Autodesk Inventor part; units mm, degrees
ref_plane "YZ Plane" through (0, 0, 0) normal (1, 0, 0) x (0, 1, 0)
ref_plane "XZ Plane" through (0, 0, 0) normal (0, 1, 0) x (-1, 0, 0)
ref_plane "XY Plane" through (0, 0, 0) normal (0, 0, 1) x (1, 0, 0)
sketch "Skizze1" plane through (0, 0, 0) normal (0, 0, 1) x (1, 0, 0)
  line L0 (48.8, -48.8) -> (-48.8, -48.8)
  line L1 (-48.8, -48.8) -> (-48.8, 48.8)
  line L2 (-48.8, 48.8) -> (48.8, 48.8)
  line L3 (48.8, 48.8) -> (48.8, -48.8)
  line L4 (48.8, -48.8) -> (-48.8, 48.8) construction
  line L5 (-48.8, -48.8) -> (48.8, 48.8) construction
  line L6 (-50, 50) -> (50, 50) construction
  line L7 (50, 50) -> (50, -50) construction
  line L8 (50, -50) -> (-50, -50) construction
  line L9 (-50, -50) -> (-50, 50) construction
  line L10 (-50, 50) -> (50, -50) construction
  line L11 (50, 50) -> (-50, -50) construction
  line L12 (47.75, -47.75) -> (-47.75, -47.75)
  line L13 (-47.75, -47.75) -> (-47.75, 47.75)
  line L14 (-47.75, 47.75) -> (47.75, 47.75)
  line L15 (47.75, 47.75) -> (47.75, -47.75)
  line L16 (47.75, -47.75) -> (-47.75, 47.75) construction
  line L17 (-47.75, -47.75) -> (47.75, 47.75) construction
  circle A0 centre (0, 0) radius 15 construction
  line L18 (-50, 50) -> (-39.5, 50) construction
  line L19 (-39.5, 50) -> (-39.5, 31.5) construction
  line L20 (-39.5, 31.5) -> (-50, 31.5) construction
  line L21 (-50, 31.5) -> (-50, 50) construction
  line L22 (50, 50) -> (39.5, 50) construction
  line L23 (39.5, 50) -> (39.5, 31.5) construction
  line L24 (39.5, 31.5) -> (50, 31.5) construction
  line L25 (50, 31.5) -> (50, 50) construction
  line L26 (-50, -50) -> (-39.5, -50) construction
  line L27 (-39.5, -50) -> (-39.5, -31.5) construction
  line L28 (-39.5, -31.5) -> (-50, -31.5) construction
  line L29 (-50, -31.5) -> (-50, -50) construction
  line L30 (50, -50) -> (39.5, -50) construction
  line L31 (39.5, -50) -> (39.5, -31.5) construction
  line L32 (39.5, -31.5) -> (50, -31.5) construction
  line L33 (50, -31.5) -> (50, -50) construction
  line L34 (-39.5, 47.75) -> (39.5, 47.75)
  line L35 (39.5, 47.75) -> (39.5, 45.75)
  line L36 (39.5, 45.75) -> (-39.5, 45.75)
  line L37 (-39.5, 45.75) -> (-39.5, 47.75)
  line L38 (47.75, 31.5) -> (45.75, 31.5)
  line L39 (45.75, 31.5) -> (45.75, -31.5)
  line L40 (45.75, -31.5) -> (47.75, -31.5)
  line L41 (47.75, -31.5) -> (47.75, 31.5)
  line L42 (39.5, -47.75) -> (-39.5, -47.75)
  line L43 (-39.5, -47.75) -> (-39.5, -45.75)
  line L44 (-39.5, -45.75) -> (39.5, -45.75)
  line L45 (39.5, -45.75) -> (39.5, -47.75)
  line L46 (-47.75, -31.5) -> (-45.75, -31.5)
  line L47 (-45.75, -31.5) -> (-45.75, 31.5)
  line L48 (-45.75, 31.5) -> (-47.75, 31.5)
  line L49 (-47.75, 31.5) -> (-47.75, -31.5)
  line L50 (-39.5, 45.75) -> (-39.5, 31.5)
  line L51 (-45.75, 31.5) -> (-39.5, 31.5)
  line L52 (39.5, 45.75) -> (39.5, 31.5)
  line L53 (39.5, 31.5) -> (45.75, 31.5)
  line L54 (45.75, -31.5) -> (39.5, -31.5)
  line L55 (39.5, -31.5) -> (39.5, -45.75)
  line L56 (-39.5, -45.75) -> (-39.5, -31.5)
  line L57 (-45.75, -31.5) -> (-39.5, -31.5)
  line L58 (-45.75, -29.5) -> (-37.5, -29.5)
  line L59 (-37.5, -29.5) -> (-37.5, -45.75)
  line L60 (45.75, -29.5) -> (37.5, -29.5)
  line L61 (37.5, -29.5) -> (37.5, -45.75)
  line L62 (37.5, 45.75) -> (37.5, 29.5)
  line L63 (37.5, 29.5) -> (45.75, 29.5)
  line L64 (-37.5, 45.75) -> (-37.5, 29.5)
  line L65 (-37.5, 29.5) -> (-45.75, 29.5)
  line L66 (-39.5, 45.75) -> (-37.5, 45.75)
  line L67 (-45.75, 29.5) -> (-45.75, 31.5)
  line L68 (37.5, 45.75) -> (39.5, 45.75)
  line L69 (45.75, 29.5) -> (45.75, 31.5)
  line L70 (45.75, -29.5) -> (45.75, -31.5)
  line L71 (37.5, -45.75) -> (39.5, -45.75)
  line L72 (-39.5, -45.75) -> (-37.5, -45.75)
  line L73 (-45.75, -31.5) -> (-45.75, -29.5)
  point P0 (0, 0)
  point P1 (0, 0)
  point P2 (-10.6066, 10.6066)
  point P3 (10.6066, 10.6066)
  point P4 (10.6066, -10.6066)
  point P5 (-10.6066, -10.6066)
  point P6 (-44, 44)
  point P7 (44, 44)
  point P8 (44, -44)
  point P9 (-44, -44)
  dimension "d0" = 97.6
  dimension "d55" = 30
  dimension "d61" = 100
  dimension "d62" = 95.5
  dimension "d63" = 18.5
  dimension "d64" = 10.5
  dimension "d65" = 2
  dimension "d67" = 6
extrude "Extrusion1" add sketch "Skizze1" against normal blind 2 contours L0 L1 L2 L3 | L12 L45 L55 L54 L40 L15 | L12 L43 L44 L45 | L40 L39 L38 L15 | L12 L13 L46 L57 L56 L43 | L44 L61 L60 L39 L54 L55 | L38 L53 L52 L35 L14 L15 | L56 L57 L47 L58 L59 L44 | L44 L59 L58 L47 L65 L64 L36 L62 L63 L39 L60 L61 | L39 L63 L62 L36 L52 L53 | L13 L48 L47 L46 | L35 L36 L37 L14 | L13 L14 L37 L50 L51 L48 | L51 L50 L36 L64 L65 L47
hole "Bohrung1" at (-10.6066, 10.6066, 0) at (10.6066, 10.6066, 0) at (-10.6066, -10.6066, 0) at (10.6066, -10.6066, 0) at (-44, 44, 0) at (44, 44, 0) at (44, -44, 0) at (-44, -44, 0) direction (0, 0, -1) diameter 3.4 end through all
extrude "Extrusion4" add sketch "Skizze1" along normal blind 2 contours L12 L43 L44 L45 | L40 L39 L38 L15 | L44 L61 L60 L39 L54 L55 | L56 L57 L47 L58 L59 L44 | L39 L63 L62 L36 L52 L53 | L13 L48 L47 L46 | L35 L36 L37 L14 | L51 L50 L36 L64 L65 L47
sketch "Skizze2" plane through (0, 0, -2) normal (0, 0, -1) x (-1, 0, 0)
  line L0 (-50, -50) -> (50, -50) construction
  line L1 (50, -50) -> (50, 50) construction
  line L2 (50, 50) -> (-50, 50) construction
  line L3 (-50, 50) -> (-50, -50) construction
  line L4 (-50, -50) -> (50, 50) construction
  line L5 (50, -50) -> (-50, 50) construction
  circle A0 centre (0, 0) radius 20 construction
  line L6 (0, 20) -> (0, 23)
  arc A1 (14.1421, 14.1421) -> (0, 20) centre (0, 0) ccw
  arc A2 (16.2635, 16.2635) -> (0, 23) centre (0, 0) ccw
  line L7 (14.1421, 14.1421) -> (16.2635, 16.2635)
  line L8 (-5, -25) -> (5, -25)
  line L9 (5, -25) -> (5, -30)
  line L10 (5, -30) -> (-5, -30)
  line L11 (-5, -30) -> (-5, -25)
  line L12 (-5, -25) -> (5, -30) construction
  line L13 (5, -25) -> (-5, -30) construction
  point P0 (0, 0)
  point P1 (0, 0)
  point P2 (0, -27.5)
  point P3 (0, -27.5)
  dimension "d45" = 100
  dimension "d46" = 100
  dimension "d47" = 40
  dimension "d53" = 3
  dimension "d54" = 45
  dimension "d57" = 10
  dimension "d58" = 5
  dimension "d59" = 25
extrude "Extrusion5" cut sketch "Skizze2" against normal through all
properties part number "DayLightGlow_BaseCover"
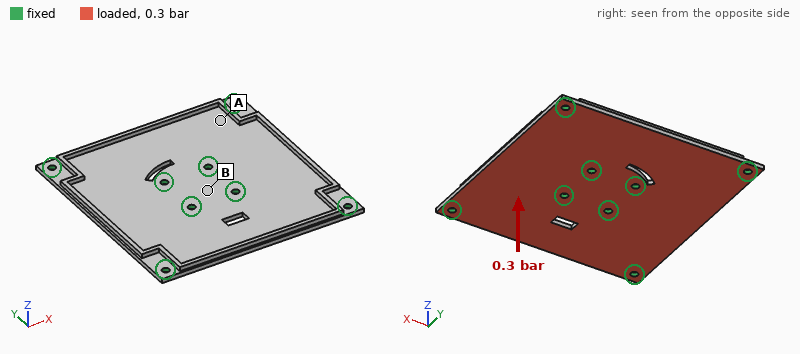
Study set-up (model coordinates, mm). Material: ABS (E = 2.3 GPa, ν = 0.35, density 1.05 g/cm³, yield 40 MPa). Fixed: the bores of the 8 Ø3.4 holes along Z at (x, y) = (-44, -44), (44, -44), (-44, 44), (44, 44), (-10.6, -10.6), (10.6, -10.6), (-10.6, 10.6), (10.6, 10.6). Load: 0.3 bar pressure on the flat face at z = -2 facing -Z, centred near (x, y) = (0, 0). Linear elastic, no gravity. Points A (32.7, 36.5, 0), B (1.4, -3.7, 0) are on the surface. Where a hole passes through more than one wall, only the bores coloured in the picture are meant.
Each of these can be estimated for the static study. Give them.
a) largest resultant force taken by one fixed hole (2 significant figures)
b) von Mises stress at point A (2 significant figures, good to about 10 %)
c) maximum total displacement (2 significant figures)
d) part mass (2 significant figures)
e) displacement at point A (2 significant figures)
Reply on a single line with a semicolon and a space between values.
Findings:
41 N; 5.3 MPa; 1.1 mm; 21 g; 0.31 mm
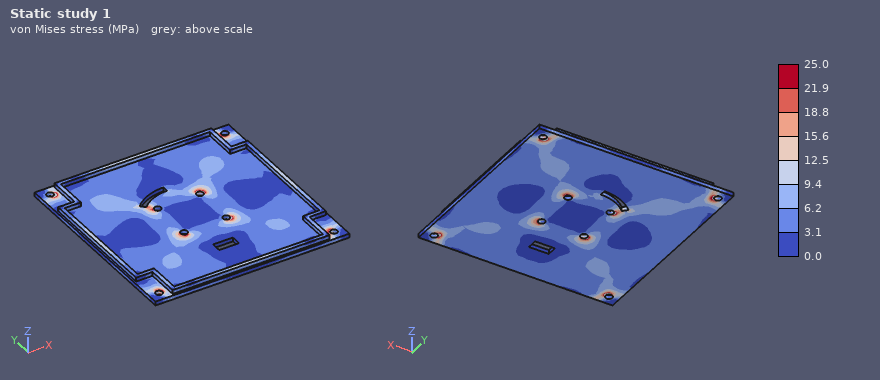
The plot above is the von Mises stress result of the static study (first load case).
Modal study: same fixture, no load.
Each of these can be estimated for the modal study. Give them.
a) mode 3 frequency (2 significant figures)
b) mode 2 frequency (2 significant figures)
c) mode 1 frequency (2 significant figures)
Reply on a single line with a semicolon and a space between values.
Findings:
690 Hz; 670 Hz; 610 Hz
